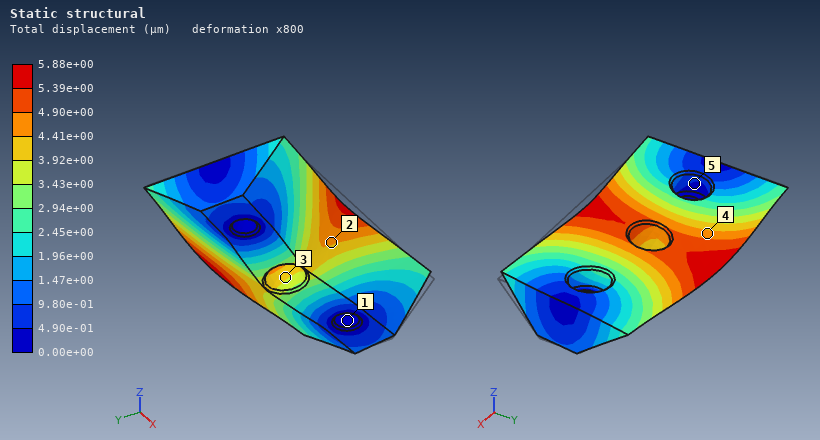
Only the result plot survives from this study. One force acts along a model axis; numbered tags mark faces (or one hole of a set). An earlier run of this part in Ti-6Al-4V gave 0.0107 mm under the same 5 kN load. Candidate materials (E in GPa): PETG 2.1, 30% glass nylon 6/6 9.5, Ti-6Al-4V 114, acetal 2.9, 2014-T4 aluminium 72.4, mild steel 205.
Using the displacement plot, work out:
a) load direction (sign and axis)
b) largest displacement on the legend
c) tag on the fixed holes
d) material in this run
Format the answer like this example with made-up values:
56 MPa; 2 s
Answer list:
+Y; 5.88e+00 µm; 1; mild steel
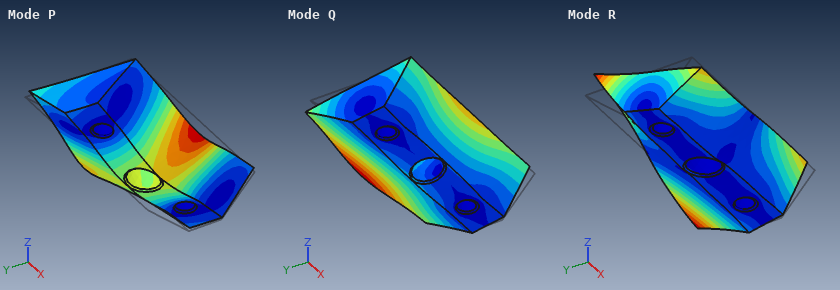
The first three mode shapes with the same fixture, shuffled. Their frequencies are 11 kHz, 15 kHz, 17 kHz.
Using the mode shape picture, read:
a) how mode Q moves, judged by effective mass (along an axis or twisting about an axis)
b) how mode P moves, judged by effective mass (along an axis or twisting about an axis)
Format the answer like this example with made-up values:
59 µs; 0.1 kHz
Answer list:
along Y; along Z
